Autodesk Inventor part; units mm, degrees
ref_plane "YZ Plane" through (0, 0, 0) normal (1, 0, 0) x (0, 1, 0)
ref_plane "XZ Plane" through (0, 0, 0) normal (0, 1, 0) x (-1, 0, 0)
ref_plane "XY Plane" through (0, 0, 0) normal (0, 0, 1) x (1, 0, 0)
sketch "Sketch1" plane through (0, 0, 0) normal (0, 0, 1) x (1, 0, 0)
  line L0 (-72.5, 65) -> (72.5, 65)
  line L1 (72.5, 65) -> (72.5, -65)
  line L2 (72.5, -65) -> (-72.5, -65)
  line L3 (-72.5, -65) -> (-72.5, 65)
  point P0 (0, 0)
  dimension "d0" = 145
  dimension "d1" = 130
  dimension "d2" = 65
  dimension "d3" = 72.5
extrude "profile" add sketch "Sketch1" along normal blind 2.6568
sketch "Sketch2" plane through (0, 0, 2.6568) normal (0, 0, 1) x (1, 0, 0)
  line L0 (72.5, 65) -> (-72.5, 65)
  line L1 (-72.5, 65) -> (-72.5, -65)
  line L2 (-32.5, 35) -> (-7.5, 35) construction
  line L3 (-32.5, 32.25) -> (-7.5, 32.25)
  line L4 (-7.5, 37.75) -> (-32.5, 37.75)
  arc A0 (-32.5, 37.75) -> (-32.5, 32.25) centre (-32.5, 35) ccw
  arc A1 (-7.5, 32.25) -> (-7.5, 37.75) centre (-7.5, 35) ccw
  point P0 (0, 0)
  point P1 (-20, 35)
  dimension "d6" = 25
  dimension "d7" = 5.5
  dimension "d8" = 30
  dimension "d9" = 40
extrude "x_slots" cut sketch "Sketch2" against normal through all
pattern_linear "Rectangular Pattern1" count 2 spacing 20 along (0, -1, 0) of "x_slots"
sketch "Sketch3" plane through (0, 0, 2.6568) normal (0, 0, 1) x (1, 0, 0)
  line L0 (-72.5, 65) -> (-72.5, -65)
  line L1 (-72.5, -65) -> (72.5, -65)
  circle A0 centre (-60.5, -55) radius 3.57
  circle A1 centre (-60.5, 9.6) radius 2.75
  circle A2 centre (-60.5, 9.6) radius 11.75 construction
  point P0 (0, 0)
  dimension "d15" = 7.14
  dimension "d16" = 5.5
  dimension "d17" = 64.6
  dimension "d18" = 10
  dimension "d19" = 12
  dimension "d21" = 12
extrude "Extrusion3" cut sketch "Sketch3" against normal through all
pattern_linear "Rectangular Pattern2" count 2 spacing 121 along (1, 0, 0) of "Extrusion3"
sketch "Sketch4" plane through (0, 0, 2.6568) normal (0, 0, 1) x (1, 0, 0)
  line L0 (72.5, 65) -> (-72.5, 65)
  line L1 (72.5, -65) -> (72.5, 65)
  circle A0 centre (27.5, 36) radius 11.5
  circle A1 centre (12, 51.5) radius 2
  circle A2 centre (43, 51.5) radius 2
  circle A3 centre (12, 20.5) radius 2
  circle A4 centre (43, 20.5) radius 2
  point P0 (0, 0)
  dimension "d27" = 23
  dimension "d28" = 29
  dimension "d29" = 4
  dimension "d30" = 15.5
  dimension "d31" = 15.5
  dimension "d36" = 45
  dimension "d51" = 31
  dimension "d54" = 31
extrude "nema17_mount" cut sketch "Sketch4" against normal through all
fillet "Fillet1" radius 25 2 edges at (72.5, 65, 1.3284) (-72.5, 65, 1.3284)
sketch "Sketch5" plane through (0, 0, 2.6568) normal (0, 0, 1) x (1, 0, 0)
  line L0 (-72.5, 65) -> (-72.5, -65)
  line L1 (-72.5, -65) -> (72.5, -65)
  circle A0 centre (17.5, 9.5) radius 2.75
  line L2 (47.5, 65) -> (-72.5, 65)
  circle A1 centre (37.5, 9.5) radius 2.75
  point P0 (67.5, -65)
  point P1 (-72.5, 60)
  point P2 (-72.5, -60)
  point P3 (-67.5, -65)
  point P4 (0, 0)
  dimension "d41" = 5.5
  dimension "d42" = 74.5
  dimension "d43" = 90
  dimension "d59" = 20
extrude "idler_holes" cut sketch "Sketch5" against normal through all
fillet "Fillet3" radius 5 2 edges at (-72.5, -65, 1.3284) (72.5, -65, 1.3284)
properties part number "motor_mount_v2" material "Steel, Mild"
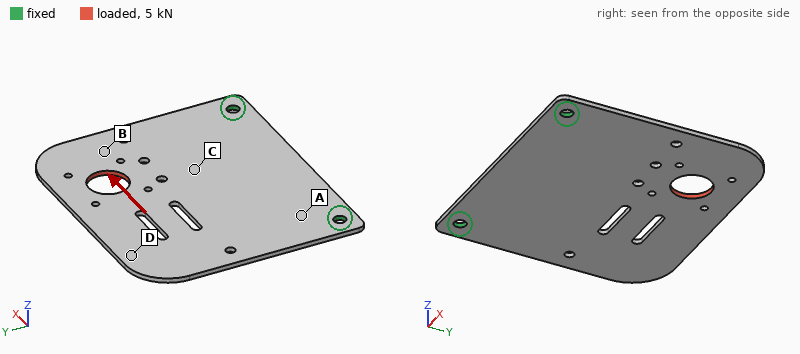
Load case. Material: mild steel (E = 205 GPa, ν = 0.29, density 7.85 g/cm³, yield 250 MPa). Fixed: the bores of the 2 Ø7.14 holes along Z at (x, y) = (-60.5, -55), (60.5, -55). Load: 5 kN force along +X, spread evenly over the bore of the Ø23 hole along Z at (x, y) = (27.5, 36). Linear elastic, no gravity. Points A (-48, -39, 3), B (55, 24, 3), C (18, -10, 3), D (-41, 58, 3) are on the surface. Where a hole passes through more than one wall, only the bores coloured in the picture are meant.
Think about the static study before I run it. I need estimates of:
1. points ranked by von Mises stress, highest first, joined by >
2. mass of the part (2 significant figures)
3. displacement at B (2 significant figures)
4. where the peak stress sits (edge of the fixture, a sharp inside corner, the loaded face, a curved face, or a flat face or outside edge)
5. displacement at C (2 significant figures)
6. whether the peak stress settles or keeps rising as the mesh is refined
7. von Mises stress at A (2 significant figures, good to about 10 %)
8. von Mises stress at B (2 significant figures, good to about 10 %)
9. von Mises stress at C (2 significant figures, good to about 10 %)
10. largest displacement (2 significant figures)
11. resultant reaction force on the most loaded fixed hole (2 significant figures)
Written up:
A > C > B > D
370 g
33 µm
edge of the fixture
15 µm
keeps rising
44 MPa
22 MPa
31 MPa
47 µm
4.5 kN
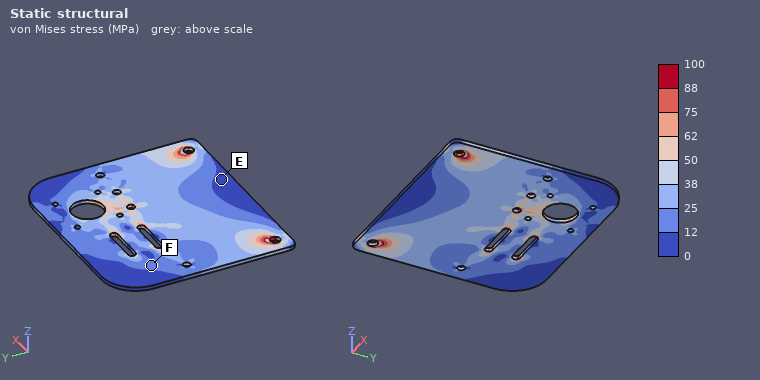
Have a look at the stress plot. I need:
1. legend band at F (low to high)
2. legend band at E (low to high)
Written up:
12 to 25 MPa
0 to 12 MPa
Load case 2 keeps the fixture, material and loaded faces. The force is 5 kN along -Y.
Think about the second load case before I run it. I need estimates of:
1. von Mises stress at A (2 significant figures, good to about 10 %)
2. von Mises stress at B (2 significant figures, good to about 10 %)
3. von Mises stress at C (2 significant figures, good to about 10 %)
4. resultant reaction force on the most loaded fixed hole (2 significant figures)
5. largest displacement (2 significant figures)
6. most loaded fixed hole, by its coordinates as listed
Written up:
18 MPa
22 MPa
15 MPa
3.7 kN
21 µm
(60.5, -55)
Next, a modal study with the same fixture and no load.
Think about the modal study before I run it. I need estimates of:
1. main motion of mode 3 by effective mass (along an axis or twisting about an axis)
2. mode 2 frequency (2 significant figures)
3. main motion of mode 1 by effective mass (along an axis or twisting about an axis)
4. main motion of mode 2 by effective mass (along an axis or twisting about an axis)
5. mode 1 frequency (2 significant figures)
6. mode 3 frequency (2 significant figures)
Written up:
along Z
350 Hz
along Z
twisting about Y
140 Hz
740 Hz
